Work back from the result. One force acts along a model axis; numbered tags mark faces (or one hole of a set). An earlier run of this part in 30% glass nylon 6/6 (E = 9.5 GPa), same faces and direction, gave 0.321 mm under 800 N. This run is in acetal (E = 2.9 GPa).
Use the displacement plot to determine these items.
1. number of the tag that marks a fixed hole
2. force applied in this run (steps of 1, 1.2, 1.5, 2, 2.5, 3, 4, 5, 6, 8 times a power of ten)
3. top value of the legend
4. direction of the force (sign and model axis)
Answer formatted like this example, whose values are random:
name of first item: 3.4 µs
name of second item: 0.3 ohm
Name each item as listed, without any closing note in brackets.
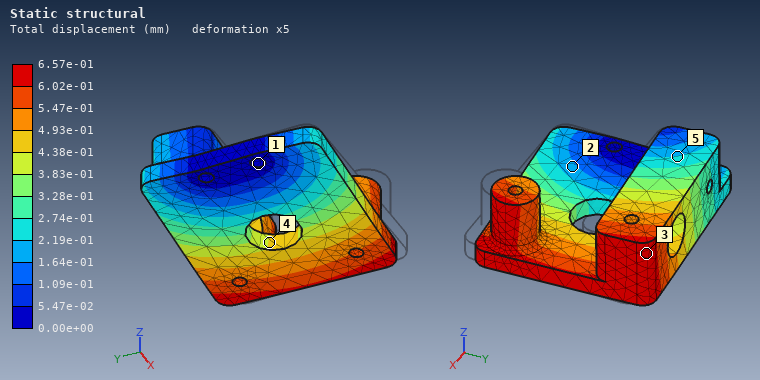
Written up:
number of the tag that marks a fixed hole: 1
force applied in this run: 500 N
top value of the legend: 6.57e-01 mm
direction of the force: +Y
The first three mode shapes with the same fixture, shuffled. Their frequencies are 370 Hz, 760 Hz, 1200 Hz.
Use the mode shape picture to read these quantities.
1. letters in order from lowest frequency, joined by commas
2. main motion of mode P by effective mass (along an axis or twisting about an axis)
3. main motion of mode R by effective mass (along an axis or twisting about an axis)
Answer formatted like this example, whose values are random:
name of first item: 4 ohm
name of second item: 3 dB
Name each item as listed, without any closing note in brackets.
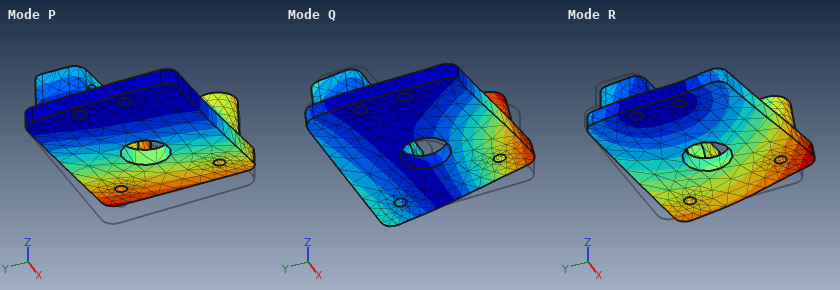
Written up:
letters in order from lowest frequency, joined by commas: P, Q, R
main motion of mode P by effective mass: along Z
main motion of mode R by effective mass: along Y
